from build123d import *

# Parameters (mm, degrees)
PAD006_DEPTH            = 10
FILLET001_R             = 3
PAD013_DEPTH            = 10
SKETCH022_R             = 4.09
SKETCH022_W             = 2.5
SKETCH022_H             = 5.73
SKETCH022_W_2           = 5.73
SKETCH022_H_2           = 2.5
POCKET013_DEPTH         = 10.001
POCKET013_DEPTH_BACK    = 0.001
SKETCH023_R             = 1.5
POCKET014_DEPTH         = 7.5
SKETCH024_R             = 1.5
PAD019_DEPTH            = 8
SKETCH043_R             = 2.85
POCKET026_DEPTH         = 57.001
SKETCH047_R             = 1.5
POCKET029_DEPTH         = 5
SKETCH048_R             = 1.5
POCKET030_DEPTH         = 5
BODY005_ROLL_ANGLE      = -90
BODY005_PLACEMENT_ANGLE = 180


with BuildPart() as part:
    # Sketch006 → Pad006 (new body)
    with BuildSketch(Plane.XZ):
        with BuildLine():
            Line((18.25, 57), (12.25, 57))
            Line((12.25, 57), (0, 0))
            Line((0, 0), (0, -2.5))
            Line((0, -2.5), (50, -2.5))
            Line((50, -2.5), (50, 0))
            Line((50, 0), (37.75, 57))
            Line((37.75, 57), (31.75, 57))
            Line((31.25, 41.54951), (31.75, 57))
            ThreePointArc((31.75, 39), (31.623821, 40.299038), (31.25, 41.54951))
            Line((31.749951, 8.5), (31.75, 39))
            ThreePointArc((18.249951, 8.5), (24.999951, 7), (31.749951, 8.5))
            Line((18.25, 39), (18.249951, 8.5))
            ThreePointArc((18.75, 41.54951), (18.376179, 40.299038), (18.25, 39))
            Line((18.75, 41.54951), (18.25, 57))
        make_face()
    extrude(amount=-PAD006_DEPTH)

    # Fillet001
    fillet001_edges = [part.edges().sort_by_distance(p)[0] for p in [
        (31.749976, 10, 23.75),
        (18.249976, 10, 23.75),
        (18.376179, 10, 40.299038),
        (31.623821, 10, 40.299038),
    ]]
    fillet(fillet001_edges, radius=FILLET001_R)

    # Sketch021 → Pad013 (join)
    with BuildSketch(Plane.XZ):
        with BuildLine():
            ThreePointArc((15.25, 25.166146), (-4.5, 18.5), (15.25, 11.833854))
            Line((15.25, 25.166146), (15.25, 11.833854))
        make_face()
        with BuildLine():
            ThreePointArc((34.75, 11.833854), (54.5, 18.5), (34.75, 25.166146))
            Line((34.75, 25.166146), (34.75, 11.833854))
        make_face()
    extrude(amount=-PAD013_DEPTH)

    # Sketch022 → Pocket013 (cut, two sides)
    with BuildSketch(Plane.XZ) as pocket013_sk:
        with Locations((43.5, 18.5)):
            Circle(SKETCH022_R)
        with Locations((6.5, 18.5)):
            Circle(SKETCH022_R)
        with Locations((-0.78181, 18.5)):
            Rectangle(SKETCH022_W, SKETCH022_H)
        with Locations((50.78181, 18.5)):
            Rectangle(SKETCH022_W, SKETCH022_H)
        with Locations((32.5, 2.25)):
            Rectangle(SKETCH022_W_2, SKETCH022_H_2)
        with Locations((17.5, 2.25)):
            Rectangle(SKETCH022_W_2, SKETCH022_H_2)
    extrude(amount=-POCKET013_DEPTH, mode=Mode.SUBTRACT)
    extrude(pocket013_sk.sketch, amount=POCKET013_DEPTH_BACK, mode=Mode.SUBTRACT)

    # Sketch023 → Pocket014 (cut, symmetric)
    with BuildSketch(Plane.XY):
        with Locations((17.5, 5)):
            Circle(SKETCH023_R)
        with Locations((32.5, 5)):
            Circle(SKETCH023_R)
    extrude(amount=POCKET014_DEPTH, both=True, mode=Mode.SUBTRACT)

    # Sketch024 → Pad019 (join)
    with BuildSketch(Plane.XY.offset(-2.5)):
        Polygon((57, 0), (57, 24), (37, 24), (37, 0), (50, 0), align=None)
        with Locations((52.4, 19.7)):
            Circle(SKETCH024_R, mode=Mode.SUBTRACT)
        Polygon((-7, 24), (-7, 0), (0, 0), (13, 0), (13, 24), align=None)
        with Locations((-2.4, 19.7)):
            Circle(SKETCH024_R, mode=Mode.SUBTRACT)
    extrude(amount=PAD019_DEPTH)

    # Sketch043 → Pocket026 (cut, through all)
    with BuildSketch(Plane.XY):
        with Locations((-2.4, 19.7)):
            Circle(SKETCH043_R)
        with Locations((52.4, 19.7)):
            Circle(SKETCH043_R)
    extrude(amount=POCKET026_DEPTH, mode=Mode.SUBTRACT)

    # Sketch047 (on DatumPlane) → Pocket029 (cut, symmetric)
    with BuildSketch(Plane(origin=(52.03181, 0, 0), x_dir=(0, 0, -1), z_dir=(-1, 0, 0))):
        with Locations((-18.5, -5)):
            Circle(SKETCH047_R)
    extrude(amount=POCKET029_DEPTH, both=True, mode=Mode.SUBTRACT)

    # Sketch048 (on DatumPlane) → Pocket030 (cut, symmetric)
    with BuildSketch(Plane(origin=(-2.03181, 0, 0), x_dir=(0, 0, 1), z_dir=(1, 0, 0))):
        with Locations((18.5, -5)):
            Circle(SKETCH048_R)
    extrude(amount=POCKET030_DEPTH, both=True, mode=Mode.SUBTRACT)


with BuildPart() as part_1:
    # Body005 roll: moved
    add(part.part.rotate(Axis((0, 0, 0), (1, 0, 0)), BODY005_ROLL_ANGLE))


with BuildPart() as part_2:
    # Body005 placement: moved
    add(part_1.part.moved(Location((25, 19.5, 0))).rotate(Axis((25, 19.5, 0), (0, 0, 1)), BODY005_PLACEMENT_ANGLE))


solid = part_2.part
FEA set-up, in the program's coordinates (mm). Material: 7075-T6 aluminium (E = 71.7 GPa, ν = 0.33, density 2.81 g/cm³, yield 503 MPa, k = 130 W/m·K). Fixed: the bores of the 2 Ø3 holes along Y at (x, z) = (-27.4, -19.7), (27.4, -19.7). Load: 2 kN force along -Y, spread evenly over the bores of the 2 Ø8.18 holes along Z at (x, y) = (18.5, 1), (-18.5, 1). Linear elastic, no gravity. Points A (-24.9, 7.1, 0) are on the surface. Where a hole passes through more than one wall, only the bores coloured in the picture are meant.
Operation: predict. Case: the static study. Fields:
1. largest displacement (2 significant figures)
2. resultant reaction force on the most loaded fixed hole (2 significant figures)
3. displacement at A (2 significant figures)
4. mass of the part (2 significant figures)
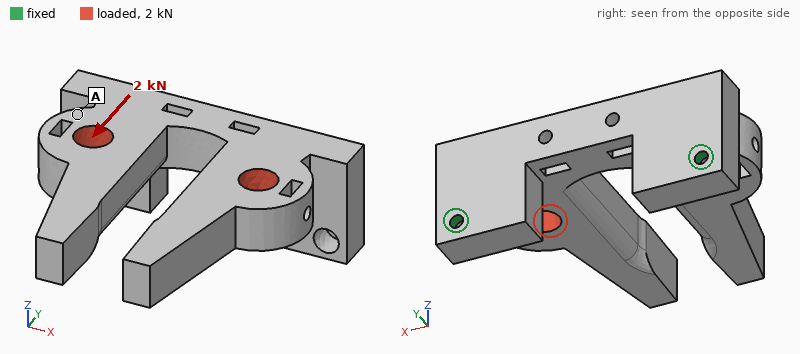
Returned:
0.88 mm
1.0 kN
0.34 mm
63 g
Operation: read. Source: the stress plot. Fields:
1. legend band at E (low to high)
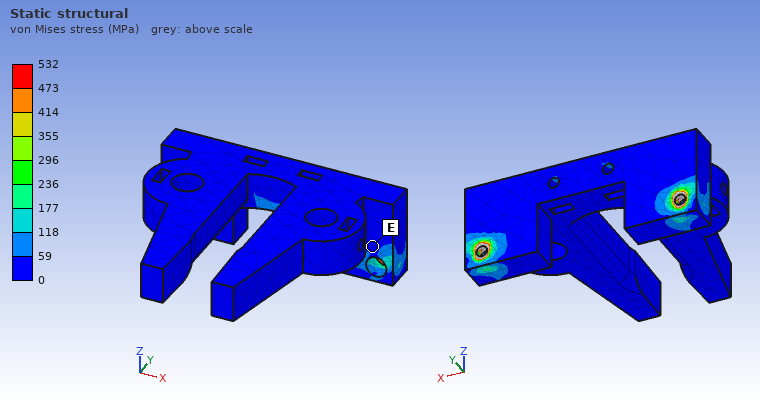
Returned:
0 to 59 MPa
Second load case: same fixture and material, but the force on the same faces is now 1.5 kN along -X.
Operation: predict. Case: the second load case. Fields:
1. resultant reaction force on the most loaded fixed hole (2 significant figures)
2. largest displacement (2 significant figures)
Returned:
980 N
0.14 mm
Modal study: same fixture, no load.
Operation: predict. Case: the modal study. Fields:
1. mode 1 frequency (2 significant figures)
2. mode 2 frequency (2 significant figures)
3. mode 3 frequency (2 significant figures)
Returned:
980 Hz
1800 Hz
2600 Hz
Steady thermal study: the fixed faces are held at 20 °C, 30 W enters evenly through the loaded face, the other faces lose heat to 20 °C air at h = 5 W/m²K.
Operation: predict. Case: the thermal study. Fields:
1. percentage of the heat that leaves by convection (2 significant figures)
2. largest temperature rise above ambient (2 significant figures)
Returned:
3.8 %
34 K
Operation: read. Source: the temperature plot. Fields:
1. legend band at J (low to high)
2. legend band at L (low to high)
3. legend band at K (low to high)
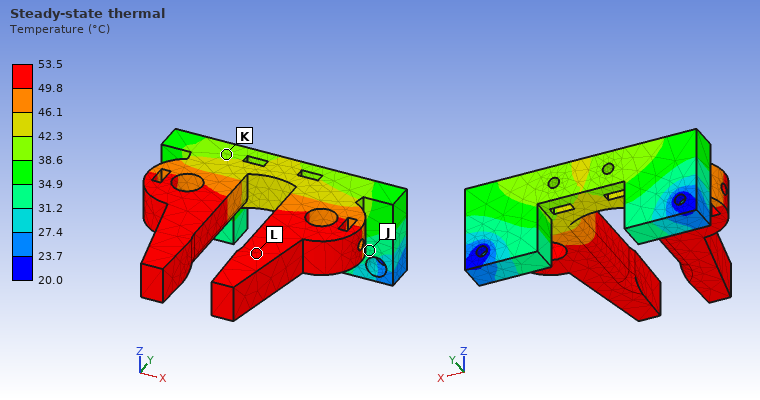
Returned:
31.2 to 34.9 °C
49.8 to 53.5 °C
38.6 to 42.3 °C
